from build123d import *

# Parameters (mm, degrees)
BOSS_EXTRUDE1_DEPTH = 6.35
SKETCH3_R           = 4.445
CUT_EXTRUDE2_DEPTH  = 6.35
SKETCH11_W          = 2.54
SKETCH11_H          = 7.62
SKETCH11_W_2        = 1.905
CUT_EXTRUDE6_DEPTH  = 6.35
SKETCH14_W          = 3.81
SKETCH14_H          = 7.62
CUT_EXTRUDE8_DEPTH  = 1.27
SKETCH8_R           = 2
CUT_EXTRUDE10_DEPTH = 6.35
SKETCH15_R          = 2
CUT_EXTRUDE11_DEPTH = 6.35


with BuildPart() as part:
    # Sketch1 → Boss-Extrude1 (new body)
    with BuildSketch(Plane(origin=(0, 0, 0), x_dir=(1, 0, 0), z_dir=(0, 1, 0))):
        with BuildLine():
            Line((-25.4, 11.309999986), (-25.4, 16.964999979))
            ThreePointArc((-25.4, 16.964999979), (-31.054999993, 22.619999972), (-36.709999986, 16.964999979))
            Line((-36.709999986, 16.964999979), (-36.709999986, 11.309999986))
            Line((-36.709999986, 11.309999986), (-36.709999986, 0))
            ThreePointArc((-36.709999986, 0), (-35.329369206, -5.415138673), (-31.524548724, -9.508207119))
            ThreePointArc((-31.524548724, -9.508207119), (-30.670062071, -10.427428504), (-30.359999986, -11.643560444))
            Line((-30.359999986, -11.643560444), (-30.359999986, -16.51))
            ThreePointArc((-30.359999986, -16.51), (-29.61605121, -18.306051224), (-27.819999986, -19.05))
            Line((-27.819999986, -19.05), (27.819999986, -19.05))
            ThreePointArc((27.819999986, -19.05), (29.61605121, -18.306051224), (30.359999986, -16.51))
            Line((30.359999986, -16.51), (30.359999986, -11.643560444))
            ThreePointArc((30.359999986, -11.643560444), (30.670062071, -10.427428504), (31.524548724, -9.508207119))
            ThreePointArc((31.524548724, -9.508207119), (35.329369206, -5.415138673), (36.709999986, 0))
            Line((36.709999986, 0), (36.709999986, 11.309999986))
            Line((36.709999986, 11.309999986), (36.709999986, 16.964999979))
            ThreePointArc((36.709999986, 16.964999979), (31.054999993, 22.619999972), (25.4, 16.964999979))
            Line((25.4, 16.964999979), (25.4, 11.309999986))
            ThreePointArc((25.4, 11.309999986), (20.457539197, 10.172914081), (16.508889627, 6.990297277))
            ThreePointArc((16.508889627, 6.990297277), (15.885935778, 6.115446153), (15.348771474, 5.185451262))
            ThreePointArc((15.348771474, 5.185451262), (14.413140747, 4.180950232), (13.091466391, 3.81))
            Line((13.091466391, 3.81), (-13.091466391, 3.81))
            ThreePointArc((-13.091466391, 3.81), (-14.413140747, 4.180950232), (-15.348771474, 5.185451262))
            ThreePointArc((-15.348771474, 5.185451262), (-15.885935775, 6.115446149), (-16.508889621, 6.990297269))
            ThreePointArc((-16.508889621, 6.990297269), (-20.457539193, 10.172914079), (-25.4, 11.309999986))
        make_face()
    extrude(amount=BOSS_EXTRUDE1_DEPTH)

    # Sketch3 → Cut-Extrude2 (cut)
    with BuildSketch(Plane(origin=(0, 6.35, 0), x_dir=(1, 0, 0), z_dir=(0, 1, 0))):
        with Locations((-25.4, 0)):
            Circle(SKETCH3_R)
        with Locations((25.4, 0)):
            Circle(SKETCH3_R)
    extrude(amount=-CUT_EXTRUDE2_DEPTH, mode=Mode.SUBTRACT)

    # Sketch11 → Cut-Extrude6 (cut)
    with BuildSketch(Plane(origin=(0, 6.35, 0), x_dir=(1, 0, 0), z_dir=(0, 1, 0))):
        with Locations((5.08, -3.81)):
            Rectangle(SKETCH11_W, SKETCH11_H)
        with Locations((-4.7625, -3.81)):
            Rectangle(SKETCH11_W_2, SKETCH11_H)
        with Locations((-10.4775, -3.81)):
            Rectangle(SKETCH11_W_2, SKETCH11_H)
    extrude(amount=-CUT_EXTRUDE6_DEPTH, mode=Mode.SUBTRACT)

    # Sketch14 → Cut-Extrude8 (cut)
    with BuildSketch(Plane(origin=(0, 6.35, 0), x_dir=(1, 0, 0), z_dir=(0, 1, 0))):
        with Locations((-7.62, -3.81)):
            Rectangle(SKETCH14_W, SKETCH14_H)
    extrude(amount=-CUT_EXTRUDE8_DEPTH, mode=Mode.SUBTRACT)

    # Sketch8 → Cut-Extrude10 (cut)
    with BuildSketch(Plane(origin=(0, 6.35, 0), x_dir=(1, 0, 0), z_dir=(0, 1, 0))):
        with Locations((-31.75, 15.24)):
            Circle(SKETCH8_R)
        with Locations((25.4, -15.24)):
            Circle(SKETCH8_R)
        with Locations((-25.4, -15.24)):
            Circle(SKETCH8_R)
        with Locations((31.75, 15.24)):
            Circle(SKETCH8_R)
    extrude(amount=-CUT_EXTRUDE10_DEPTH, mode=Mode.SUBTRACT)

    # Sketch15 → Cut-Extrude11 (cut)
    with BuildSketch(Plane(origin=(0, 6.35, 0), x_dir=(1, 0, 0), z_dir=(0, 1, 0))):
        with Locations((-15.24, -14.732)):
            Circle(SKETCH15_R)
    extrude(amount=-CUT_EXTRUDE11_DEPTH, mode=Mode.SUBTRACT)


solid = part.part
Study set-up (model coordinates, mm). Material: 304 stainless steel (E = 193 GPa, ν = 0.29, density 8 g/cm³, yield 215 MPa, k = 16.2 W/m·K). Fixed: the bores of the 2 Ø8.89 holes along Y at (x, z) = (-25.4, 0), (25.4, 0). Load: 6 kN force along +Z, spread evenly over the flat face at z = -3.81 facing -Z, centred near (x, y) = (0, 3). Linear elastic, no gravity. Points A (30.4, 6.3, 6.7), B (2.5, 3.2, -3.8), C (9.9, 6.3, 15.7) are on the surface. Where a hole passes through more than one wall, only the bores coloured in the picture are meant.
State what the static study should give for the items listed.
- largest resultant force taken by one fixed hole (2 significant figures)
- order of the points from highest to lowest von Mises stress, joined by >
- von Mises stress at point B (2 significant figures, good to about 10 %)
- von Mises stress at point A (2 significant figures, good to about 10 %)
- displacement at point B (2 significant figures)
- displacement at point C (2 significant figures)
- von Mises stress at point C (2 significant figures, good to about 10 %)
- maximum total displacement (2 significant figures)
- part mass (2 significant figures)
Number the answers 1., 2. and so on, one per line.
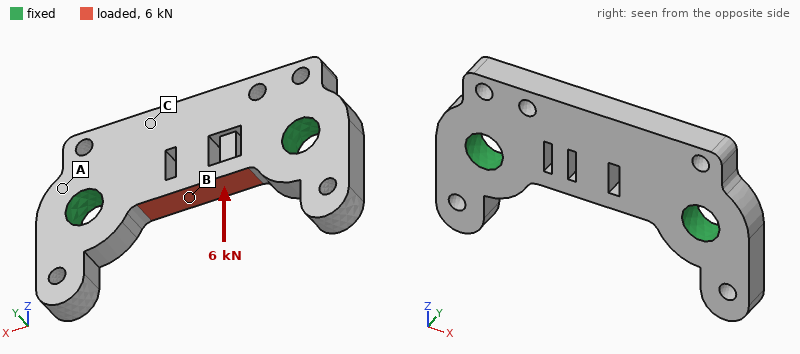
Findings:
1. 3.3 kN
2. B > C > A
3. 48 MPa
4. 11 MPa
5. 11 µm
6. 6.6 µm
7. 31 MPa
8. 12 µm
9. 91 g
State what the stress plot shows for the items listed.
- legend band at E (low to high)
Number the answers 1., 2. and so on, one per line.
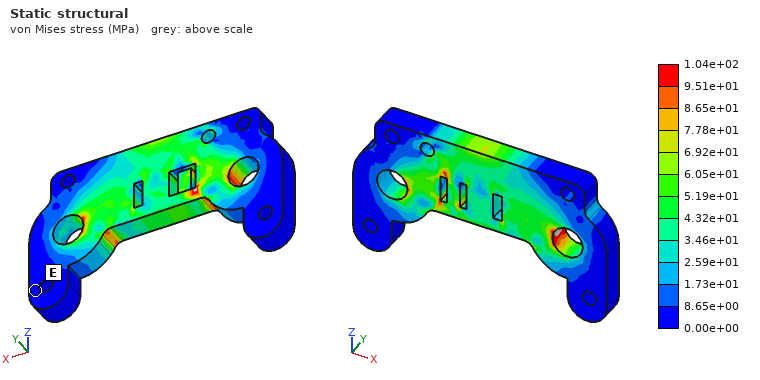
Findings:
1. 0.00e+00 to 8.65e+00 MPa
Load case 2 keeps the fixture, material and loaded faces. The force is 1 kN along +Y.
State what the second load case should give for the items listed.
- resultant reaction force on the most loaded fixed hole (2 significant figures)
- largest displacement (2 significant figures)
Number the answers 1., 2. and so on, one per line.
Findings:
1. 500 N
2. 12 µm
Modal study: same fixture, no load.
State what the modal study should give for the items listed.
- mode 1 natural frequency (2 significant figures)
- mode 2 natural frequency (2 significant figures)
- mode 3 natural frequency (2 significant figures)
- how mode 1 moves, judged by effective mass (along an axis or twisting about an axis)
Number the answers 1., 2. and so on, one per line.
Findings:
1. 10000 Hz
2. 15 kHz
3. 15 kHz
4. along Y
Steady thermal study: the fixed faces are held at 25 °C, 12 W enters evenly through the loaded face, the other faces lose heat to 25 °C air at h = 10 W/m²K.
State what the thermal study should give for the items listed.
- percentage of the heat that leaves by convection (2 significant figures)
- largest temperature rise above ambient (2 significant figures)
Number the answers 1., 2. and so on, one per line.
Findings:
1. 7.7 %
2. 82 K
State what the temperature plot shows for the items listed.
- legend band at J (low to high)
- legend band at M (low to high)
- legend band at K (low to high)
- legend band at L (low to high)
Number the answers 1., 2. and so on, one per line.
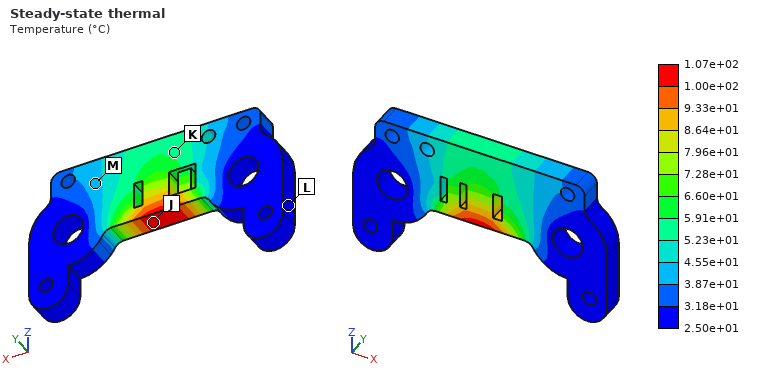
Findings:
1. 1.00e+02 to 1.07e+02 °C
2. 3.87e+01 to 4.55e+01 °C
3. 5.23e+01 to 5.91e+01 °C
4. 2.50e+01 to 3.18e+01 °C
